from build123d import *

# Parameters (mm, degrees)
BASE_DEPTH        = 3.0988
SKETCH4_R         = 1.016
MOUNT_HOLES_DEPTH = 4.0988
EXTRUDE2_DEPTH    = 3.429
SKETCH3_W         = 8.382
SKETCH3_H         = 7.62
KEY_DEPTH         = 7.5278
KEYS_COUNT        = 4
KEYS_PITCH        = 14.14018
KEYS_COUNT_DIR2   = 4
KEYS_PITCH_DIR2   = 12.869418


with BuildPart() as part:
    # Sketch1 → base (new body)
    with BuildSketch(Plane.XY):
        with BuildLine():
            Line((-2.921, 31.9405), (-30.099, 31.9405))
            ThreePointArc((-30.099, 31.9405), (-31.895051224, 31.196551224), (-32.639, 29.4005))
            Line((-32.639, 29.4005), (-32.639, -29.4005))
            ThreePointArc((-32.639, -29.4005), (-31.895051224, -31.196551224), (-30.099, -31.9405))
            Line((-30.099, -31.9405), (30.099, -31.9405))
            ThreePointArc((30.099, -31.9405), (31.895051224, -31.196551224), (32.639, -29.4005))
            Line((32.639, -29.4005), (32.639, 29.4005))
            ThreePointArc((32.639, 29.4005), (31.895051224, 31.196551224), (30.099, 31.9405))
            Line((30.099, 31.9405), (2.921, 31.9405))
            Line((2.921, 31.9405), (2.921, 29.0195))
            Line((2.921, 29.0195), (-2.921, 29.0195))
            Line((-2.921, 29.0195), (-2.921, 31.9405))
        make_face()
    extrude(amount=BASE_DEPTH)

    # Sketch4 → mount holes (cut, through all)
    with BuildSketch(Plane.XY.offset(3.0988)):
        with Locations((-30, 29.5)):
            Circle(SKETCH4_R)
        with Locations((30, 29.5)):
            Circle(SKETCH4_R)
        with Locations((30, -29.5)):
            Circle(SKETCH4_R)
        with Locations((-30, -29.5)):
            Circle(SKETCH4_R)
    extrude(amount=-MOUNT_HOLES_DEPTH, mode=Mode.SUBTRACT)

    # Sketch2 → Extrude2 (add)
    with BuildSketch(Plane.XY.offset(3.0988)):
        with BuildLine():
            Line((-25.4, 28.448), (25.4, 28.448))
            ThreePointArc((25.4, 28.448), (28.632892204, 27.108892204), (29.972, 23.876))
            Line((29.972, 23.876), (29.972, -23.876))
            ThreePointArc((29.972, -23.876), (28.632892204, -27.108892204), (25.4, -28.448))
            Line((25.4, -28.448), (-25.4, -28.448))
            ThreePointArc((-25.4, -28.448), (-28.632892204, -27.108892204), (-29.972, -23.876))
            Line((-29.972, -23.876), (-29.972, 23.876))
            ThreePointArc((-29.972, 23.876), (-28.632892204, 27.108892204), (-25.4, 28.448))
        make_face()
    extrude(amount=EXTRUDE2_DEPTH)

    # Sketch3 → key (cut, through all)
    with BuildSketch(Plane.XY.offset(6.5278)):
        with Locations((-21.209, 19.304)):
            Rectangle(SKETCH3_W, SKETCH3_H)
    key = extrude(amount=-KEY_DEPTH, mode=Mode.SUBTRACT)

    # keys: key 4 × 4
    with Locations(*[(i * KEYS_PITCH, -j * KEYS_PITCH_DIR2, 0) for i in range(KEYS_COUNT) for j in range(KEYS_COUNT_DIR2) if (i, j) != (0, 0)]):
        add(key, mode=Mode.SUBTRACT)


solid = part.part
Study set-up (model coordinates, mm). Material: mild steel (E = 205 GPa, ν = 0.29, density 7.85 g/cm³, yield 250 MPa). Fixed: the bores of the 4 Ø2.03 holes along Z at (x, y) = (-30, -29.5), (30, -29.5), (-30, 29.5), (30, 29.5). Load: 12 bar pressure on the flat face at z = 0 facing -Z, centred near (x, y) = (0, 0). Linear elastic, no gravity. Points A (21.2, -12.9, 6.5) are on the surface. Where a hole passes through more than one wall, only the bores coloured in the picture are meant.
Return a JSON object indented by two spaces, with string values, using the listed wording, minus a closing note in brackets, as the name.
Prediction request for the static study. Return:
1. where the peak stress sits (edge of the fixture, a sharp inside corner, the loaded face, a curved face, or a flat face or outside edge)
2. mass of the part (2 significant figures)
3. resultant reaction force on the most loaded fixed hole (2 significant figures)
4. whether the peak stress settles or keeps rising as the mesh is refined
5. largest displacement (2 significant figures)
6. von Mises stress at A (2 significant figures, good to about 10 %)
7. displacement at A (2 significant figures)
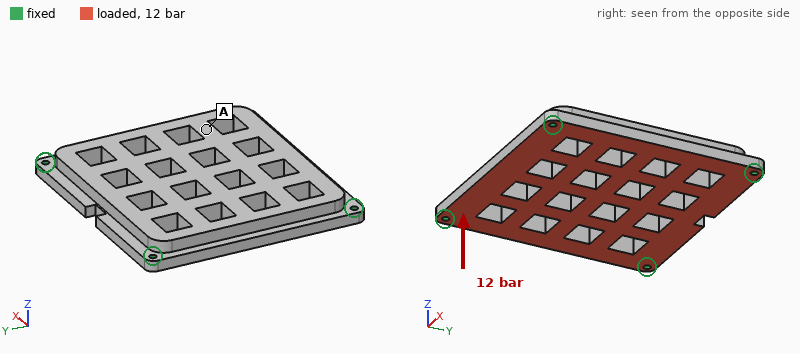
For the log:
{
  "where the peak stress sits": "edge of the fixture",
  "mass of the part": "140 g",
  "resultant reaction force on the most loaded fixed hole": "1.5 kN",
  "whether the peak stress settles or keeps rising as the mesh is refined": "keeps rising",
  "largest displacement": "63 µm",
  "von Mises stress at A": "47 MPa",
  "displacement at A": "42 µm"
}
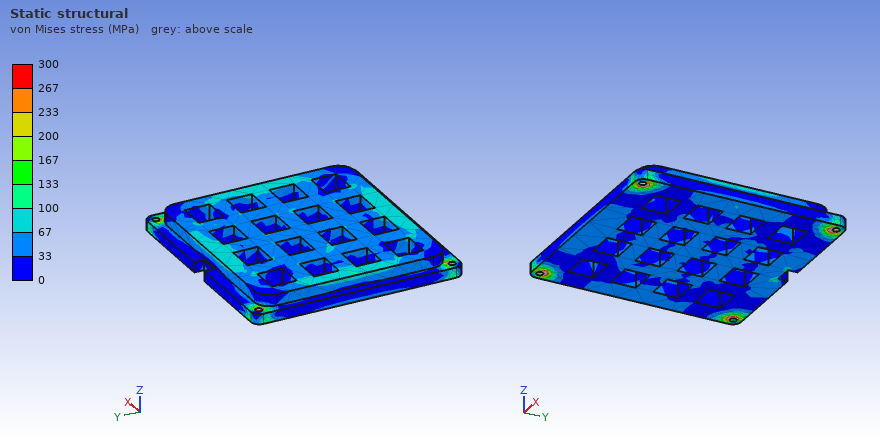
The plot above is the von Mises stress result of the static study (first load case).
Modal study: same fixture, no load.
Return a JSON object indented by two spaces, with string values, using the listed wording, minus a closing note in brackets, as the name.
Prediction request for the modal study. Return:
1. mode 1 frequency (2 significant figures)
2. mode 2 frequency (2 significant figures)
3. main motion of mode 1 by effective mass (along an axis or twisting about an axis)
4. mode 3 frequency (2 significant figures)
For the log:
{
  "mode 1 frequency": "3700 Hz",
  "mode 2 frequency": "6400 Hz",
  "main motion of mode 1 by effective mass": "along Z",
  "mode 3 frequency": "6600 Hz"
}
